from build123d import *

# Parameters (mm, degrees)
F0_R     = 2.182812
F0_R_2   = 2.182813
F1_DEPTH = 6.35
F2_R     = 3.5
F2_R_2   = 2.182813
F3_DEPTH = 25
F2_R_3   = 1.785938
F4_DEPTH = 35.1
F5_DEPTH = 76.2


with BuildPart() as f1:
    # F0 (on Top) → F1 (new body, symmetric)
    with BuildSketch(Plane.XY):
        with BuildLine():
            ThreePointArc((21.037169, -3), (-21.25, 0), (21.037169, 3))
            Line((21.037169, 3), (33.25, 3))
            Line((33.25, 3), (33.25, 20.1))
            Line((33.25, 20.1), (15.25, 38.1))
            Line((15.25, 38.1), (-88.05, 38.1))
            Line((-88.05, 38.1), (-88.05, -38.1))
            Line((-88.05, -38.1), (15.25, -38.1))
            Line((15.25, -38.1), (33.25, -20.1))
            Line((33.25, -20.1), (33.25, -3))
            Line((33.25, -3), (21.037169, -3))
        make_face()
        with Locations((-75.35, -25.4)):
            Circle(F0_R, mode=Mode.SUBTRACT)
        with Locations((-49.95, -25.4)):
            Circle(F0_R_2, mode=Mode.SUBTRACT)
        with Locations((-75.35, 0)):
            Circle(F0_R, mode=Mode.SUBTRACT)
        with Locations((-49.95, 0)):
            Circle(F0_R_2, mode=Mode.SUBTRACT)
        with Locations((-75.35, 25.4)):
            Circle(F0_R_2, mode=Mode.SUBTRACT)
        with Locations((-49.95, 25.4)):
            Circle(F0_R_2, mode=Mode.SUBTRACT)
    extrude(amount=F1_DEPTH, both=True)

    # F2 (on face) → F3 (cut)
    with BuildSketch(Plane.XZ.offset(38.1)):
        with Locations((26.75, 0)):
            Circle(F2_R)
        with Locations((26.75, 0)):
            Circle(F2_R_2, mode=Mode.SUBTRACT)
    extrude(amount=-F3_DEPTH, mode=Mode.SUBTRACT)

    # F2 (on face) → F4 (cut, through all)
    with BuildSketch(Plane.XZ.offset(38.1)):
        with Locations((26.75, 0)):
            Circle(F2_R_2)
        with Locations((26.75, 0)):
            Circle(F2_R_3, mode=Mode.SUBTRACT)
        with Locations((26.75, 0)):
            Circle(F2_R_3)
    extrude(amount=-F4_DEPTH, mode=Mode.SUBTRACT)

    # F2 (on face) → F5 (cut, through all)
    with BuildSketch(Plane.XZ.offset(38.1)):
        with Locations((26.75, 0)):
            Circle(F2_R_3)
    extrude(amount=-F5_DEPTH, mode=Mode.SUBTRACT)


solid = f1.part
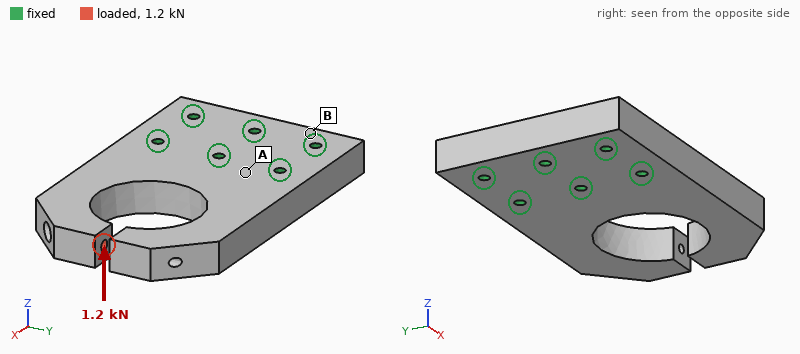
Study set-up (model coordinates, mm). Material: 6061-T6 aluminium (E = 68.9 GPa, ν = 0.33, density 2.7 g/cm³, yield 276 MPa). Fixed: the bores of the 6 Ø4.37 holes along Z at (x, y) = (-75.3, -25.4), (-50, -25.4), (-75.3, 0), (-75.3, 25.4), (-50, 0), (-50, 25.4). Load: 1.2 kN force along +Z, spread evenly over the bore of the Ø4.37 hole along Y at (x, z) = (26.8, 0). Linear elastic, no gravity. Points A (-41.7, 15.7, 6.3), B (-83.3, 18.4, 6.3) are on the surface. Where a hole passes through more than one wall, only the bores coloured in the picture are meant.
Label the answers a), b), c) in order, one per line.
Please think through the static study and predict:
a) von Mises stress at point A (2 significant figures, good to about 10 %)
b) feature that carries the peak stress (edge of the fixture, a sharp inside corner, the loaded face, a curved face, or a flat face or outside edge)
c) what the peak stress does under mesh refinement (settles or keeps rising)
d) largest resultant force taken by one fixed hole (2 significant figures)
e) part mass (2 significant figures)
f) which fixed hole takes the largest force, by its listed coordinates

a) 23 MPa
b) edge of the fixture
c) keeps rising
d) 1.5 kN
e) 250 g
f) (-50, 0)
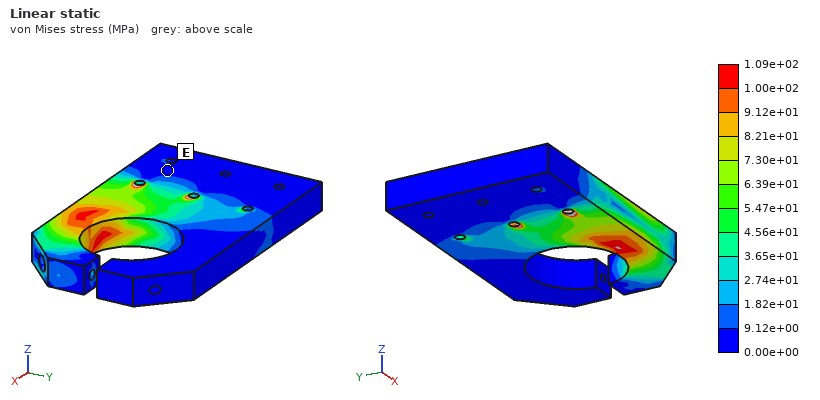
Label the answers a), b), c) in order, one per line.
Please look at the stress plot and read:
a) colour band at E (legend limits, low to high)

a) 0.00e+00 to 9.12e+00 MPa
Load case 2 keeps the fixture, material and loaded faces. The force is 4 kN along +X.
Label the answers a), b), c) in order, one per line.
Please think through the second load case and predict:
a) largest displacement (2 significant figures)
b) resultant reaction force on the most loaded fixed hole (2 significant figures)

a) 0.40 mm
b) 1.7 kN
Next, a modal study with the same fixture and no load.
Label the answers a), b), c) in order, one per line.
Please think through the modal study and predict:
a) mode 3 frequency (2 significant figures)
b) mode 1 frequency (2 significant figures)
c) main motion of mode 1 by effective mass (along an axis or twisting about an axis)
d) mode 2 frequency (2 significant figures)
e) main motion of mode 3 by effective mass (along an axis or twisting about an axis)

a) 3700 Hz
b) 1700 Hz
c) along Z
d) 1900 Hz
e) along Y
